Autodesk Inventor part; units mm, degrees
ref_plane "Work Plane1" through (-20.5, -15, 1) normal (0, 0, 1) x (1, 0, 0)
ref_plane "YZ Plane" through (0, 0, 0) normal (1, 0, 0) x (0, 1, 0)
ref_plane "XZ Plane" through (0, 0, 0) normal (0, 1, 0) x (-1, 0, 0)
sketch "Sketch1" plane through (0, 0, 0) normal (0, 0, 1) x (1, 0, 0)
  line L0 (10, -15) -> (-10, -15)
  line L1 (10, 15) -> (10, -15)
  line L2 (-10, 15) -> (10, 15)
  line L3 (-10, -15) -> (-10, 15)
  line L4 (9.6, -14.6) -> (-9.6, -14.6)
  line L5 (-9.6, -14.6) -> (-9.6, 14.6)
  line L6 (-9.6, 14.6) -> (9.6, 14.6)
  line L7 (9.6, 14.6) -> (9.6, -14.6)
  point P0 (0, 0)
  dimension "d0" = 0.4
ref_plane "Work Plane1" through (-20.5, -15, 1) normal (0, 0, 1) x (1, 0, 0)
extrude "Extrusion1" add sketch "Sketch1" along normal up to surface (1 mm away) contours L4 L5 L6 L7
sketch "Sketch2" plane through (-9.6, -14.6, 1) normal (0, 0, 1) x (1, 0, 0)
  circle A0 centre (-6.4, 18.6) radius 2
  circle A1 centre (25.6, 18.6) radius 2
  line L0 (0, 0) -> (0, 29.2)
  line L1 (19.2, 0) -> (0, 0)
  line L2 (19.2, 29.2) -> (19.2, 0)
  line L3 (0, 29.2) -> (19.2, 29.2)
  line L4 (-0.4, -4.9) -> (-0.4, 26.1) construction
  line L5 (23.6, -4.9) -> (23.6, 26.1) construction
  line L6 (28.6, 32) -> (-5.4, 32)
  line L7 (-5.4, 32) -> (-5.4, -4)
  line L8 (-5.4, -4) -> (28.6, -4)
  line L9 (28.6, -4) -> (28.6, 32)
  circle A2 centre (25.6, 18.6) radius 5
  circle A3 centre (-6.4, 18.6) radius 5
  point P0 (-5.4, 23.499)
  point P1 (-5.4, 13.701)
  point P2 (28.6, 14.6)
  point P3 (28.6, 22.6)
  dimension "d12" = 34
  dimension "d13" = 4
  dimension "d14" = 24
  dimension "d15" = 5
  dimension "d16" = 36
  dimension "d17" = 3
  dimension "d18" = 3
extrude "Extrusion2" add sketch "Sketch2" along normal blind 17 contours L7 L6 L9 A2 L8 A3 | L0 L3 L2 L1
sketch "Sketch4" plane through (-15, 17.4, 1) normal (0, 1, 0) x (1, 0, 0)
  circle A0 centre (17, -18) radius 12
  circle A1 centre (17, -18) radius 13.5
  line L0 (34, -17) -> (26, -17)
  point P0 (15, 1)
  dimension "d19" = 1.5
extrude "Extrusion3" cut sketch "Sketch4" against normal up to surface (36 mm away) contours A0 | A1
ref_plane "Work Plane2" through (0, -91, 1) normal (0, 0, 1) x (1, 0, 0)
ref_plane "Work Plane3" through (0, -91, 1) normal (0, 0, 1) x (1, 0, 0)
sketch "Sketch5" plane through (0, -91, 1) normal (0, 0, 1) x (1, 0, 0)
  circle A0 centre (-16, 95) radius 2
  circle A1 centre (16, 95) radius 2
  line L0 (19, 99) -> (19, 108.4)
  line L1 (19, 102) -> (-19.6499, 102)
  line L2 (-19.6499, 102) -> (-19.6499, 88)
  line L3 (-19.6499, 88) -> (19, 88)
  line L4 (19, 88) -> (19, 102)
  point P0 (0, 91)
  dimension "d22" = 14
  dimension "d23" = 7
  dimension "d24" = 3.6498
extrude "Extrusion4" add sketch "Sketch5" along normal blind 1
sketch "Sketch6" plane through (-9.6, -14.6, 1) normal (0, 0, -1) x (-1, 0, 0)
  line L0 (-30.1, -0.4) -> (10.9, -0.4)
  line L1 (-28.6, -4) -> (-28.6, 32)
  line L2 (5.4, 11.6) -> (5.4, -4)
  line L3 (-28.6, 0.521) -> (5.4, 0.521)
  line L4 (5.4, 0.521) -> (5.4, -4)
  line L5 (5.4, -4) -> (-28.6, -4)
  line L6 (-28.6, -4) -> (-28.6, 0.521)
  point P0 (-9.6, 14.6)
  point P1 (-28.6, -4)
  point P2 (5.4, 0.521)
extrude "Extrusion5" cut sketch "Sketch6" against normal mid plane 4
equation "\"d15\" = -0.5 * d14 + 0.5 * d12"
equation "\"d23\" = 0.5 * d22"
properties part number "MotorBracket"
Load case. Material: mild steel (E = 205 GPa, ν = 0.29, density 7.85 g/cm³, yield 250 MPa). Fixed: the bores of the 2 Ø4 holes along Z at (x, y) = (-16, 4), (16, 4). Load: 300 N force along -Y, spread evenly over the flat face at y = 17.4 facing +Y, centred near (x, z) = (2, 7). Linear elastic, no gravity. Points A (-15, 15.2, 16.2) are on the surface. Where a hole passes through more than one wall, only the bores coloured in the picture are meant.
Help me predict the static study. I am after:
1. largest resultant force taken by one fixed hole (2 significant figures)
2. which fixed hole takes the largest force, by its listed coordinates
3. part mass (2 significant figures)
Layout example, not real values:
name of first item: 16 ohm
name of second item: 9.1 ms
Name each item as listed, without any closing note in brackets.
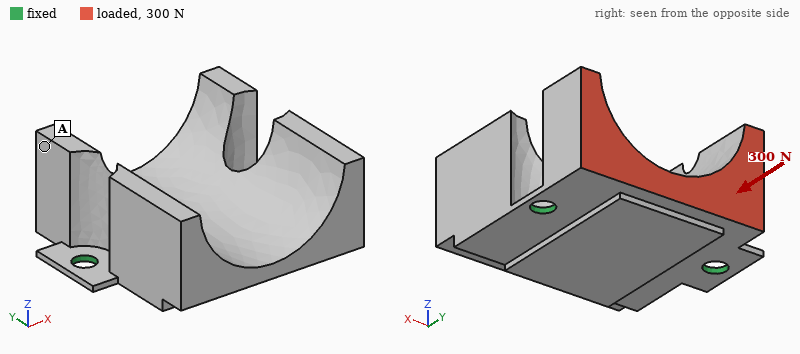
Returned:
largest resultant force taken by one fixed hole: 170 N
which fixed hole takes the largest force, by its listed coordinates: (16, 4)
part mass: 82 g
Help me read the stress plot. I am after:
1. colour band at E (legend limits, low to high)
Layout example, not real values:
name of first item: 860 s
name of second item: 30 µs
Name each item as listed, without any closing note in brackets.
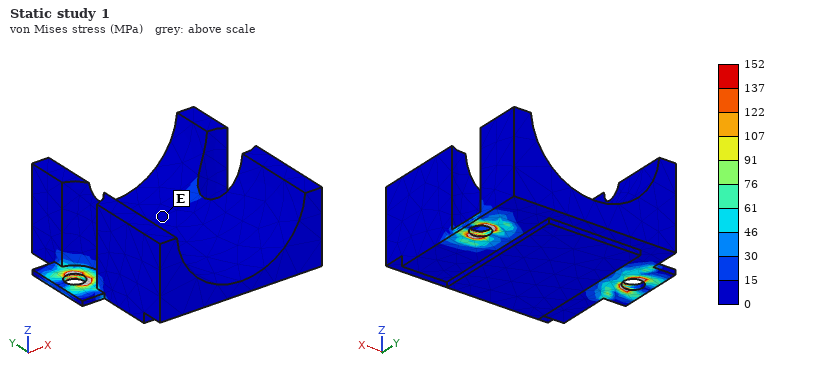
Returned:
colour band at E: 0 to 15 MPa
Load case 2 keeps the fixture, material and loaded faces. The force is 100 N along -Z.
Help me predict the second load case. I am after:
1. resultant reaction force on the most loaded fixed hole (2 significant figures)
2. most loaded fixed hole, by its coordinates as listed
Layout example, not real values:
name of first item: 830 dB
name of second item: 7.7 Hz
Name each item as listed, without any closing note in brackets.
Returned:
resultant reaction force on the most loaded fixed hole: 62 N
most loaded fixed hole, by its coordinates as listed: (16, 4)
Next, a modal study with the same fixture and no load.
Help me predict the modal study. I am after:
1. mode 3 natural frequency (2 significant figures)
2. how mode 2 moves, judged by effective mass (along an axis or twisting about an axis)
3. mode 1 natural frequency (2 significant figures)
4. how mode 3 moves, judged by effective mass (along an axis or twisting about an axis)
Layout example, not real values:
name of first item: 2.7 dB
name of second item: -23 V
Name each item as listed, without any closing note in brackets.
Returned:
mode 3 natural frequency: 6500 Hz
how mode 2 moves, judged by effective mass: along Z
mode 1 natural frequency: 1300 Hz
how mode 3 moves, judged by effective mass: along Z
